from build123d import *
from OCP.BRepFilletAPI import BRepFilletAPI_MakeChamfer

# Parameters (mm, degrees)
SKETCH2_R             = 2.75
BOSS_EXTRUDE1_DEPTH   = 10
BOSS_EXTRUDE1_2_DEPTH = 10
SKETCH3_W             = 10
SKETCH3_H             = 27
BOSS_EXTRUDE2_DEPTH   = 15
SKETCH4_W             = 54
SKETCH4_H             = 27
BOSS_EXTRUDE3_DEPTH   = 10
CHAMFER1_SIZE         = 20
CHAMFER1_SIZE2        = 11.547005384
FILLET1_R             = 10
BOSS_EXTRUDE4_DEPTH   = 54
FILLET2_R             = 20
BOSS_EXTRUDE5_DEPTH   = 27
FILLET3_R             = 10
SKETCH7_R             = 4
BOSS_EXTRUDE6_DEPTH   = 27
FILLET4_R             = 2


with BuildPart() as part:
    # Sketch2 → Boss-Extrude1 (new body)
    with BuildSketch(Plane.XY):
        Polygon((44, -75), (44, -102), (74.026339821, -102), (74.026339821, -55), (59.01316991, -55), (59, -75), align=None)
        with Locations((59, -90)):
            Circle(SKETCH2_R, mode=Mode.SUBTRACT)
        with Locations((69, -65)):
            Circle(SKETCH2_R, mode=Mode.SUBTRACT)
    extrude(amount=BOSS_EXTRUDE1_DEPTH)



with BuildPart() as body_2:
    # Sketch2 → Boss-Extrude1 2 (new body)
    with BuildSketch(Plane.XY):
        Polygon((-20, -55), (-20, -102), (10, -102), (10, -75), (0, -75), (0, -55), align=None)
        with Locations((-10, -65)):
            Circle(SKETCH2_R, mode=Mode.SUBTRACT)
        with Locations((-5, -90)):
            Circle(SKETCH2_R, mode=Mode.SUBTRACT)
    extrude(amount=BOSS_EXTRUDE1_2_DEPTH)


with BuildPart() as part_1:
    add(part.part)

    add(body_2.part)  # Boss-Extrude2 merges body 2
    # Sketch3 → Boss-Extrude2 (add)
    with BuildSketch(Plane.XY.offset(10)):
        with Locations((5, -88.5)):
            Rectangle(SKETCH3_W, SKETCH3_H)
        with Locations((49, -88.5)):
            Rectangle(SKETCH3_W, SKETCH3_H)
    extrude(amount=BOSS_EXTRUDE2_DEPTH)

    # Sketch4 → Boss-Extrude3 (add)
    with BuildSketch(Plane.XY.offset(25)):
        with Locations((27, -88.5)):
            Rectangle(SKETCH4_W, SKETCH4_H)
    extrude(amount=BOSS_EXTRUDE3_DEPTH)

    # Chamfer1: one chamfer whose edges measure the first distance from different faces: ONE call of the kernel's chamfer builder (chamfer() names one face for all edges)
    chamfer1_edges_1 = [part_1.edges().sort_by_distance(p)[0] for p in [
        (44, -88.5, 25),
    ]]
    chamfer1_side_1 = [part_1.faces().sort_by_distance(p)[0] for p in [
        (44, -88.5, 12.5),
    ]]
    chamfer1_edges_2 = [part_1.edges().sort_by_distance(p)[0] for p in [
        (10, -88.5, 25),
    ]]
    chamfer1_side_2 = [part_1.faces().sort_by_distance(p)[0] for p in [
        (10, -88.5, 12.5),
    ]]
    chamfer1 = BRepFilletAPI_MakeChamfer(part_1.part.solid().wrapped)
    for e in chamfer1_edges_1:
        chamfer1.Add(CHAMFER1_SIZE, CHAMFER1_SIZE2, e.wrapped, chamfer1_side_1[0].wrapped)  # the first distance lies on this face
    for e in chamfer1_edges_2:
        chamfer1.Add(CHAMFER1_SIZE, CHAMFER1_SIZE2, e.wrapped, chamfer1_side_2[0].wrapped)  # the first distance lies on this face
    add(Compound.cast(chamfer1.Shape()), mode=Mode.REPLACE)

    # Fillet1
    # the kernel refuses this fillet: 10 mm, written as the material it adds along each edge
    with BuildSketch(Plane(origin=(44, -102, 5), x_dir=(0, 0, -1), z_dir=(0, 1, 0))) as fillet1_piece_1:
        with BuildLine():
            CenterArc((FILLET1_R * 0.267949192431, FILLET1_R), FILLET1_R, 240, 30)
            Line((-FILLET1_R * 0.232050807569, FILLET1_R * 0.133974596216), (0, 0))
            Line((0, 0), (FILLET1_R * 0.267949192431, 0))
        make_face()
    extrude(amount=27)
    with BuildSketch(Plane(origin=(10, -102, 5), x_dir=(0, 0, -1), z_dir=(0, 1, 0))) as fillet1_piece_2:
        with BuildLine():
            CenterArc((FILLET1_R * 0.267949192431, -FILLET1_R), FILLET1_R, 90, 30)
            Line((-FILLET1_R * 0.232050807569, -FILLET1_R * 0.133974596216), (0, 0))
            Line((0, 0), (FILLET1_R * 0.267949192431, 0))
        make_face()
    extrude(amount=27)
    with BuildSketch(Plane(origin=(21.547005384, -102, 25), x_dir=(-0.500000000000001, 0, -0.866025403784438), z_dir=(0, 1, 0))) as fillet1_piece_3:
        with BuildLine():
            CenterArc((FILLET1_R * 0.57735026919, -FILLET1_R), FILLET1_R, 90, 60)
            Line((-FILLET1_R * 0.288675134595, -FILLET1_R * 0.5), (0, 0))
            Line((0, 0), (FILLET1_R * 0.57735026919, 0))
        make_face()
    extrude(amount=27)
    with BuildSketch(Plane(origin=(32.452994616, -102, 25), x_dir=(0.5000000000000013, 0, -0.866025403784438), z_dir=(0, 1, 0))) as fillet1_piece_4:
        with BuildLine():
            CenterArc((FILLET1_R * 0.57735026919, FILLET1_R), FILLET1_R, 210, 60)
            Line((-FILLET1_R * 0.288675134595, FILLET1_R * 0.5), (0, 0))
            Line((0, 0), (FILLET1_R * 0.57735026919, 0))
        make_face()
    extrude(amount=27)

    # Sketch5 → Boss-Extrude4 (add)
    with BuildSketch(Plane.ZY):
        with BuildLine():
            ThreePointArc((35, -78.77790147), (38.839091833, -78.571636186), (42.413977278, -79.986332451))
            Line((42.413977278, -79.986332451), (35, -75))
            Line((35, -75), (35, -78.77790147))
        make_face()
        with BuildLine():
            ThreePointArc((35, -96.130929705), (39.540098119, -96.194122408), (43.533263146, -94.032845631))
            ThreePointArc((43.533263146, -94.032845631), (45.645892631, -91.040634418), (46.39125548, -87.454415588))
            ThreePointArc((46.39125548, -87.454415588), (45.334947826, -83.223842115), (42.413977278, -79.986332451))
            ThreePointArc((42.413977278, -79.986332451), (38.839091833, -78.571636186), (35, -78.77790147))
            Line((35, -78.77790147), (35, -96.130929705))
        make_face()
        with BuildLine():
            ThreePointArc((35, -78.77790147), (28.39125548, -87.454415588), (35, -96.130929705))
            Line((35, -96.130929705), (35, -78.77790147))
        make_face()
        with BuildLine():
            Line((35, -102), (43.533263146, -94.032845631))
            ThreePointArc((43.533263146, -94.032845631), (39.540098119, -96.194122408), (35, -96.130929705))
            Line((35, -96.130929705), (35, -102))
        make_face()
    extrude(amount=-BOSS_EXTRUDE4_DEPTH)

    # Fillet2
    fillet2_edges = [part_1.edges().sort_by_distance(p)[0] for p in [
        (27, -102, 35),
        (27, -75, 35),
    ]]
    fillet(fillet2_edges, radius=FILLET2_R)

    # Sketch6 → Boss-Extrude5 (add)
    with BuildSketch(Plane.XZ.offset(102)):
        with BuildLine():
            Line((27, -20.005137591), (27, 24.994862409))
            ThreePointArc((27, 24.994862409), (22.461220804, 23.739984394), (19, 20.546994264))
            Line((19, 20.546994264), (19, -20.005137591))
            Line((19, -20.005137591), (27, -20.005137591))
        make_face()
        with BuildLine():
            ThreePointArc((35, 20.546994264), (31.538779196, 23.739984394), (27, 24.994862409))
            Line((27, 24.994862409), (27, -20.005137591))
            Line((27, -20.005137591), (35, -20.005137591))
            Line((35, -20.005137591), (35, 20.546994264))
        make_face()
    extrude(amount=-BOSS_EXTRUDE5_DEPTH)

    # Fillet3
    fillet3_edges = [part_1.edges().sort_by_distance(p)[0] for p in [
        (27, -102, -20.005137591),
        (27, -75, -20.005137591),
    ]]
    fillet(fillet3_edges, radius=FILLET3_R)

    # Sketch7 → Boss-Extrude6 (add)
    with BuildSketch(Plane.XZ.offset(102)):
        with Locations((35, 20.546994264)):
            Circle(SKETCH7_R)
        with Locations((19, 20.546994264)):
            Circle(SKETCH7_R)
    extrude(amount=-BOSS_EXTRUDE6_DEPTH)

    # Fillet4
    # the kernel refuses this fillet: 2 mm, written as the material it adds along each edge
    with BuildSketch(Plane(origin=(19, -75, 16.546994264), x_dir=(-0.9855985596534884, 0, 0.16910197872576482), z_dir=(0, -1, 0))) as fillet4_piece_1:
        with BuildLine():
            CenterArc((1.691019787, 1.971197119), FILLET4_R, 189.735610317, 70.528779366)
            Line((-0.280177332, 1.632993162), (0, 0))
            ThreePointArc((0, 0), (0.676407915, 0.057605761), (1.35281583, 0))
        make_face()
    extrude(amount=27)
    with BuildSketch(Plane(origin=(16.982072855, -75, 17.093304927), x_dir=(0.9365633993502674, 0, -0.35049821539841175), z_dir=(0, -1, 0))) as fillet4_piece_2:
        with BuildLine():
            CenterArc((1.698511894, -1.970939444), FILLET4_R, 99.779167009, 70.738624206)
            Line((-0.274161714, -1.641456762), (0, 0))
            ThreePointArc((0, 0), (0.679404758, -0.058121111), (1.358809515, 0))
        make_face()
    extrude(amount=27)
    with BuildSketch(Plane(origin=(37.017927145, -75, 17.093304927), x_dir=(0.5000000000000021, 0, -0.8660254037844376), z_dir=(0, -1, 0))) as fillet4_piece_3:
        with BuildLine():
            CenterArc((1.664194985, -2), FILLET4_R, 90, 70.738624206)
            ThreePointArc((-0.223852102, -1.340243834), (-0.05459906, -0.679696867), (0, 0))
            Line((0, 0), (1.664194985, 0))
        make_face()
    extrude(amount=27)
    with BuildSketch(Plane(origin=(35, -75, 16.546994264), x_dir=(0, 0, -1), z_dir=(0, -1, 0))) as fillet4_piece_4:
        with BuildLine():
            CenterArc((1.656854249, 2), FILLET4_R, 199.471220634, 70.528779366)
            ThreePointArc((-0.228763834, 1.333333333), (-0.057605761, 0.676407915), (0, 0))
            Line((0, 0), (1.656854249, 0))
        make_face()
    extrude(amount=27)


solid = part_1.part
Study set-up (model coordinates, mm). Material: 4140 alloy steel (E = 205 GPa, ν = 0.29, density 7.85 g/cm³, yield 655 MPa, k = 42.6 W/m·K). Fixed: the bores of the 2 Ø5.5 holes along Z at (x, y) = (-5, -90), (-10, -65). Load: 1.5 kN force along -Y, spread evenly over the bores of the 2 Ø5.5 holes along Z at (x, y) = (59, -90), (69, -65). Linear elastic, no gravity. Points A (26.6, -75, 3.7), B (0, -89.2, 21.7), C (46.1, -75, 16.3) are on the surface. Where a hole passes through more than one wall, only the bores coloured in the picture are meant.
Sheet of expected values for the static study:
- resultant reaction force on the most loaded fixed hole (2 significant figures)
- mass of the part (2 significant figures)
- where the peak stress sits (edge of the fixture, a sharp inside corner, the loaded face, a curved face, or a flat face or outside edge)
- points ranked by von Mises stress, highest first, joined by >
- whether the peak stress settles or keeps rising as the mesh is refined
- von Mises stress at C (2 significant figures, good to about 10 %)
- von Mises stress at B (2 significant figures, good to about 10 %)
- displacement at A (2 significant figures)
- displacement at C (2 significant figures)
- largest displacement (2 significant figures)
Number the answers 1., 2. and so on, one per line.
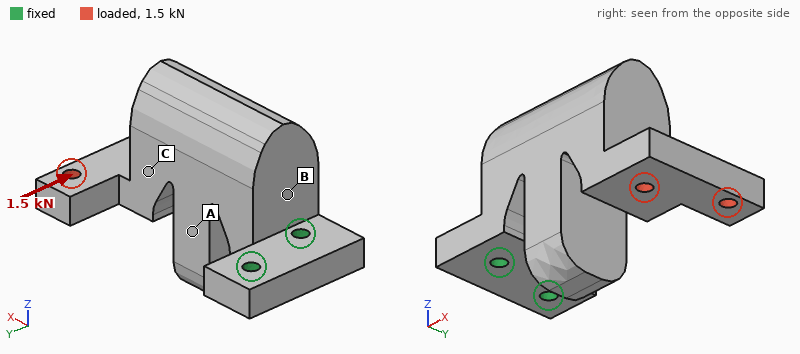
1. 3.7 kN
2. 630 g
3. edge of the fixture
4. B > C > A
5. keeps rising
6. 23 MPa
7. 46 MPa
8. 0.043 mm
9. 0.066 mm
10. 0.14 mm
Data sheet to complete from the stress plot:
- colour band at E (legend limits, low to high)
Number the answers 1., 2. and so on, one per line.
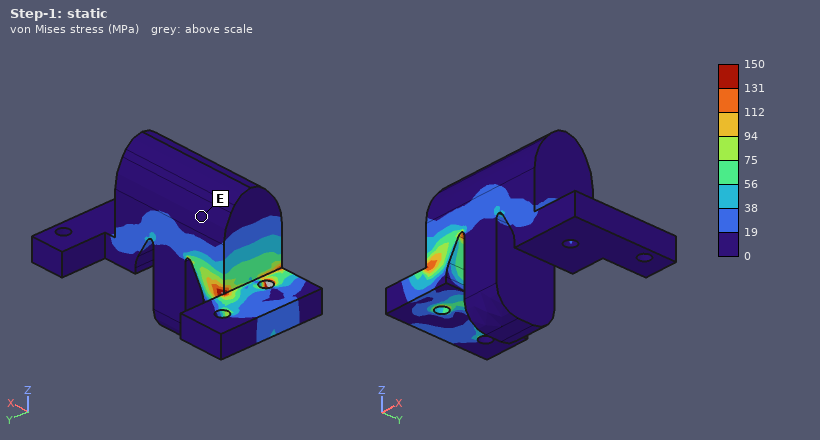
1. 0 to 19 MPa
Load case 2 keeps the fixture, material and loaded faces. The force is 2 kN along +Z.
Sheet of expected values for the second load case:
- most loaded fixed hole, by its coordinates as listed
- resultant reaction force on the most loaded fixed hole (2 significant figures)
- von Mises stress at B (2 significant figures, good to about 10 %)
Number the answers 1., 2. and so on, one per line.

1. (-5, -90)
2. 2.1 kN
3. 61 MPa
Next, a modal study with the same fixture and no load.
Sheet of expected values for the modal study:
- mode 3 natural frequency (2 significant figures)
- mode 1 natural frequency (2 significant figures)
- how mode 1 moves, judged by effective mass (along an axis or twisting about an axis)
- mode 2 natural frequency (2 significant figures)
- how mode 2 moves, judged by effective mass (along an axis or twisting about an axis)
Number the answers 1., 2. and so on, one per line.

1. 2800 Hz
2. 900 Hz
3. along Z
4. 1500 Hz
5. along Y
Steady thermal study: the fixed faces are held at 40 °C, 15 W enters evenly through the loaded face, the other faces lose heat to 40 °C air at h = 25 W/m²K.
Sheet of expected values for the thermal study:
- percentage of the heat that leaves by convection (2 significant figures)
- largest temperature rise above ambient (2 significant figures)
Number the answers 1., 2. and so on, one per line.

1. 54 %
2. 63 K
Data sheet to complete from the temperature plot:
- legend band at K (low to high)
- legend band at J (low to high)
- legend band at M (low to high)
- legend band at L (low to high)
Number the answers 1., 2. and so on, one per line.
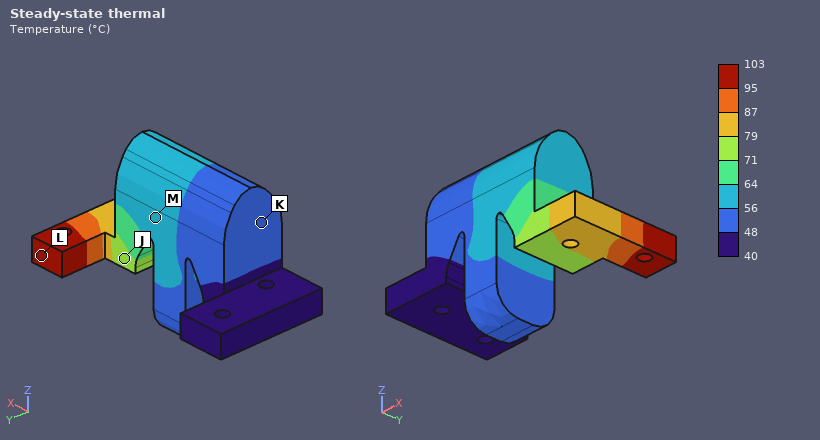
1. 48 to 56 °C
2. 71 to 79 °C
3. 56 to 64 °C
4. 95 to 103 °C
